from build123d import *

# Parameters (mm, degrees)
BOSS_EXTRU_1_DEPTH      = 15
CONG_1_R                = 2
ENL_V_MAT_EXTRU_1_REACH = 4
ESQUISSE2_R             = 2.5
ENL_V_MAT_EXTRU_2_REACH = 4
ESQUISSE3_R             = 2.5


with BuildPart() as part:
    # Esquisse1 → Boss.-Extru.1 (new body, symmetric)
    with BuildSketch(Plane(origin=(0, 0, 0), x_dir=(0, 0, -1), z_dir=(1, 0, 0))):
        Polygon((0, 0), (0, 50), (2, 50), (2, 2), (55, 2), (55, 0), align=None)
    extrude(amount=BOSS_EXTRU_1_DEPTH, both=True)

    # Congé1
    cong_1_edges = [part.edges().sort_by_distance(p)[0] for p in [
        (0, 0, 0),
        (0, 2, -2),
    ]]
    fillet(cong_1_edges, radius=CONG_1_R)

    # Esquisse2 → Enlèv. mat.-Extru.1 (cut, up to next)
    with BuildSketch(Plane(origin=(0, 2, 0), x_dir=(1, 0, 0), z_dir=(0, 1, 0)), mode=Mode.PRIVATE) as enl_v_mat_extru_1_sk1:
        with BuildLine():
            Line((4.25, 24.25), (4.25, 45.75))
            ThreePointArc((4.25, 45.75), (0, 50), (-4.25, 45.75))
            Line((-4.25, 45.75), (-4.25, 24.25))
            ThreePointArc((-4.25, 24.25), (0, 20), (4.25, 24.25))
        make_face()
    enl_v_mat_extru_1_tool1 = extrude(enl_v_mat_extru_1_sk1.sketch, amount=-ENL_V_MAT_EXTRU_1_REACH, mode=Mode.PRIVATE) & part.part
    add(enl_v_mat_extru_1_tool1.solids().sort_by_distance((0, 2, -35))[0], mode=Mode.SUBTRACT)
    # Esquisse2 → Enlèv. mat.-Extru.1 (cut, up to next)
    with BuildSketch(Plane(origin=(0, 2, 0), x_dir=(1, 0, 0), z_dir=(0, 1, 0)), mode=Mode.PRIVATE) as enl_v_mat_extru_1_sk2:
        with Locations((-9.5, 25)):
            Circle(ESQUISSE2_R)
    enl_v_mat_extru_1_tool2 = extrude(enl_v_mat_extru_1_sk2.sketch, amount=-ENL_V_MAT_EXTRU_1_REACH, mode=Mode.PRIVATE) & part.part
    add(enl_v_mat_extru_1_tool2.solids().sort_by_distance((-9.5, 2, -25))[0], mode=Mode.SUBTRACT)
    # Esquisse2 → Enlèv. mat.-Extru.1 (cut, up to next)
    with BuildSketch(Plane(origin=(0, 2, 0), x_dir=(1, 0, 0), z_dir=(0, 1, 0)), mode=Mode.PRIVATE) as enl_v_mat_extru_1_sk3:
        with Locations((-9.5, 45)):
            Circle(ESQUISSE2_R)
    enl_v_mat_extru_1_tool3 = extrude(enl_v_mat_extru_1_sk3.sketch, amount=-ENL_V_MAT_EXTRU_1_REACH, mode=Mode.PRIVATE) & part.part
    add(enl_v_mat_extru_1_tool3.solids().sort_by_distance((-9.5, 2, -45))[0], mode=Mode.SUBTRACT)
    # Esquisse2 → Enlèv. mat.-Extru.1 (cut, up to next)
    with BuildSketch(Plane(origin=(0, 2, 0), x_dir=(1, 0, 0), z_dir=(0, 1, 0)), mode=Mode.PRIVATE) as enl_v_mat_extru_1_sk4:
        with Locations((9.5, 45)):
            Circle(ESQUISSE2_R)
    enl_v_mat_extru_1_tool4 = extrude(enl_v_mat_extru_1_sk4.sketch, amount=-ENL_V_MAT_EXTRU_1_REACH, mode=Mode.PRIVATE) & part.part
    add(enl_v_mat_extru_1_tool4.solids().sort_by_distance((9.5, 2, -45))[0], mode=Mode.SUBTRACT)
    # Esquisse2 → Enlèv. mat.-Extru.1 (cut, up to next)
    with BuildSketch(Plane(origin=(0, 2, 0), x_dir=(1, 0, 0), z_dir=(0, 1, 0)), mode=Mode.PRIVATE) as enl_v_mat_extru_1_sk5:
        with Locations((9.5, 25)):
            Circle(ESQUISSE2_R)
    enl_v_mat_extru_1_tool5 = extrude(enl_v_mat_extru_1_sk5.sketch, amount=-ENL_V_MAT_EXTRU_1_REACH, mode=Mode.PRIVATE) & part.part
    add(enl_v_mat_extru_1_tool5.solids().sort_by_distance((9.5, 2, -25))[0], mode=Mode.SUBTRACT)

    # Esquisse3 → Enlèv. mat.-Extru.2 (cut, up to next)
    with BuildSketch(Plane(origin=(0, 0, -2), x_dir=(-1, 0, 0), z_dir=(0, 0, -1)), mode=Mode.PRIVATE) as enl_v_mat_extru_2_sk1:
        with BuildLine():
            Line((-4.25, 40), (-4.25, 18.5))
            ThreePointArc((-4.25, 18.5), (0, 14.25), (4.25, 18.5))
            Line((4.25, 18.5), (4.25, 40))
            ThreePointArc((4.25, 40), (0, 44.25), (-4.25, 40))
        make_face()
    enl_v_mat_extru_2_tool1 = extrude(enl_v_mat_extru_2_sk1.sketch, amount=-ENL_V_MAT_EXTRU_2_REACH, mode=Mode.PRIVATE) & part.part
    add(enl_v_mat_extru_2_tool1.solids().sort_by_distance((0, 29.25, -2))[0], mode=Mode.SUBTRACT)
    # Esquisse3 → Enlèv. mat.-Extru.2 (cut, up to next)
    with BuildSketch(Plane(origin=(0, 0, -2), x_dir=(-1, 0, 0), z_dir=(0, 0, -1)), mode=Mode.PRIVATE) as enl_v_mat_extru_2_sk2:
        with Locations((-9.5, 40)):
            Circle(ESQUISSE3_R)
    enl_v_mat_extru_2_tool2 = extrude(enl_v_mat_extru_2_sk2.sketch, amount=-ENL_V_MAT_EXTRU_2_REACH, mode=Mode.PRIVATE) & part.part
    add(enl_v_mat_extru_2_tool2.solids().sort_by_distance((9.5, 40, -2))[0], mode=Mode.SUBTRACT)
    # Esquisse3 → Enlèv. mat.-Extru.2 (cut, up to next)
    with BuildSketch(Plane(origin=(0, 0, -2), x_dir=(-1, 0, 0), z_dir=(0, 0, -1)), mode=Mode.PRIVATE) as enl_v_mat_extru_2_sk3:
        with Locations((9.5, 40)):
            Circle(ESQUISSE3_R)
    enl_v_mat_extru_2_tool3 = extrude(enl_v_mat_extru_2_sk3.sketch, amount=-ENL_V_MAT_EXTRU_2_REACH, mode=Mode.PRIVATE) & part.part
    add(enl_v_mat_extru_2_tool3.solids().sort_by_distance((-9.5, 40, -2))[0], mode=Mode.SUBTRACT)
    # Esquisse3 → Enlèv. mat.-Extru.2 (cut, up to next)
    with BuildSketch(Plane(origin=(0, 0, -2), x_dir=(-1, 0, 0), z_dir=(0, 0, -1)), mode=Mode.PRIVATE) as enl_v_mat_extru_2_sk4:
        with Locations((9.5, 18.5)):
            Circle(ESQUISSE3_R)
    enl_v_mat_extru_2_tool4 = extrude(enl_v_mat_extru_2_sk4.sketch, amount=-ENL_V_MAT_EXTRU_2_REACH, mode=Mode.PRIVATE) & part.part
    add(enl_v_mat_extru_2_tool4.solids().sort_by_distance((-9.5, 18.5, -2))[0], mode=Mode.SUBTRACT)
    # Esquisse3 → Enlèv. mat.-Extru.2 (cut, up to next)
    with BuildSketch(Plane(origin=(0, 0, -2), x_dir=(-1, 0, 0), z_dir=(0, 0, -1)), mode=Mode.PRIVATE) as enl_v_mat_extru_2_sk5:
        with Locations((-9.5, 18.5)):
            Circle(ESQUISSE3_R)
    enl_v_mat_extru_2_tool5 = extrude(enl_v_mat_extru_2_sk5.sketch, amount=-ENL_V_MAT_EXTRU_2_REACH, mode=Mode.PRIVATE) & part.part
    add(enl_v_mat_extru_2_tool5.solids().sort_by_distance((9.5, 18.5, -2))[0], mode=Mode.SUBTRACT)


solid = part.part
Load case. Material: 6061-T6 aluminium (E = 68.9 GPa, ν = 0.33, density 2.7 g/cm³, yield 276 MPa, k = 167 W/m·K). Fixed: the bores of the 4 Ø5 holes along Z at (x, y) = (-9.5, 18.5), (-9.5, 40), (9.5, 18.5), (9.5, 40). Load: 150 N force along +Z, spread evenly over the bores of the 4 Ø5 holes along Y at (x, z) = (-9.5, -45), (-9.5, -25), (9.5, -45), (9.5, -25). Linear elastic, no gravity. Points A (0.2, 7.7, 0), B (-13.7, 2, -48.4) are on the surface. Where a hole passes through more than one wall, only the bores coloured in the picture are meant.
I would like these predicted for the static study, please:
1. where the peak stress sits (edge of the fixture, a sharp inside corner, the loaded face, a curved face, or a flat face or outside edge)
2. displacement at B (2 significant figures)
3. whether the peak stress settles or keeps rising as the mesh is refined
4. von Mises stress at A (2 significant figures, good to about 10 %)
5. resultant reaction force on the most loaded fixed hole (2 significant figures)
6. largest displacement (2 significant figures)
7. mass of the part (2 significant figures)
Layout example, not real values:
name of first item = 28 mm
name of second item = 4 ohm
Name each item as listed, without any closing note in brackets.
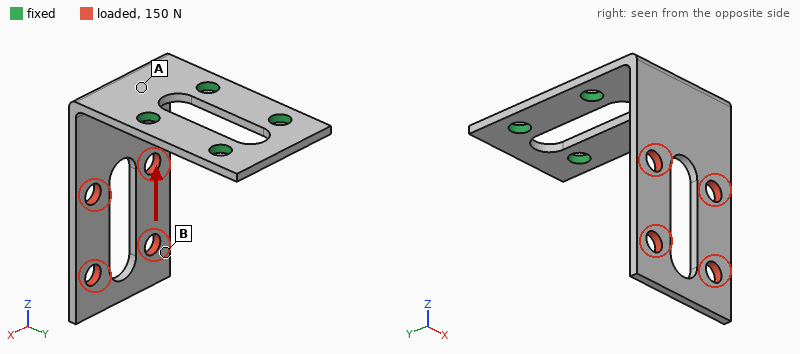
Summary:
where the peak stress sits = edge of the fixture
displacement at B = 0.69 mm
whether the peak stress settles or keeps rising as the mesh is refined = keeps rising
von Mises stress at A = 41 MPa
resultant reaction force on the most loaded fixed hole = 75 N
largest displacement = 0.79 mm
mass of the part = 13 g
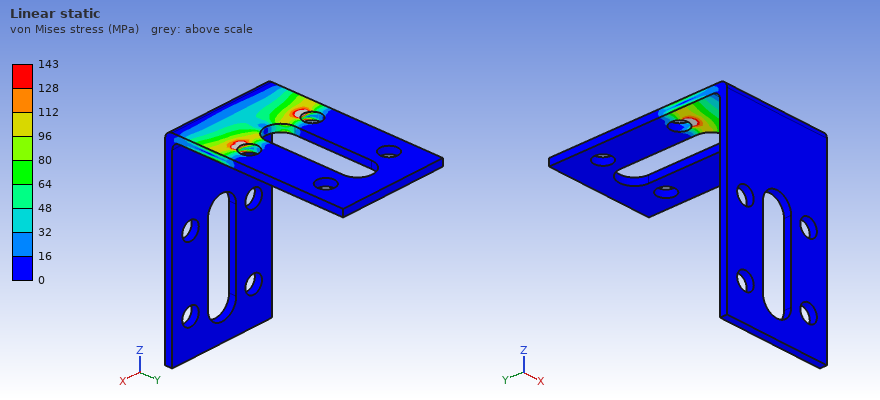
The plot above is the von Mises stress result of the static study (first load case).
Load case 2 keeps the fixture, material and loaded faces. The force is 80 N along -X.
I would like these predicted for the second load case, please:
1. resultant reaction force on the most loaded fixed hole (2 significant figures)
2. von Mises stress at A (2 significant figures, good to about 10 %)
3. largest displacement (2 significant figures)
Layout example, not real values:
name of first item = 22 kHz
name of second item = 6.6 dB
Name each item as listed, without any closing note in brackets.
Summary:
resultant reaction force on the most loaded fixed hole = 140 N
von Mises stress at A = 56 MPa
largest displacement = 0.48 mm
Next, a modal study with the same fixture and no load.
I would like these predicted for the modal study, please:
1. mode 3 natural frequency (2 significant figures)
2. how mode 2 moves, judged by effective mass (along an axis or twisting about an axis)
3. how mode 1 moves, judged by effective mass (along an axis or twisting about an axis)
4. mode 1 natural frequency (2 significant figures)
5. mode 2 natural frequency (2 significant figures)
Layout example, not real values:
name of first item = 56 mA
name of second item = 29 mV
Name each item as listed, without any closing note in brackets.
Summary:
mode 3 natural frequency = 1900 Hz
how mode 2 moves, judged by effective mass = along X
how mode 1 moves, judged by effective mass = along Y
mode 1 natural frequency = 440 Hz
mode 2 natural frequency = 1100 Hz
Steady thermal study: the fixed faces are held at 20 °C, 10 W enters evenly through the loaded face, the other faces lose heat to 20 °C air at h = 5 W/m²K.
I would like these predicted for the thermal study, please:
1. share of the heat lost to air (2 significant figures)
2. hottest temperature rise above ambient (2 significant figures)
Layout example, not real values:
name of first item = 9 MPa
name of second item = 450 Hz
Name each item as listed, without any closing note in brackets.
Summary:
share of the heat lost to air = 6.5 %
hottest temperature rise above ambient = 59 K
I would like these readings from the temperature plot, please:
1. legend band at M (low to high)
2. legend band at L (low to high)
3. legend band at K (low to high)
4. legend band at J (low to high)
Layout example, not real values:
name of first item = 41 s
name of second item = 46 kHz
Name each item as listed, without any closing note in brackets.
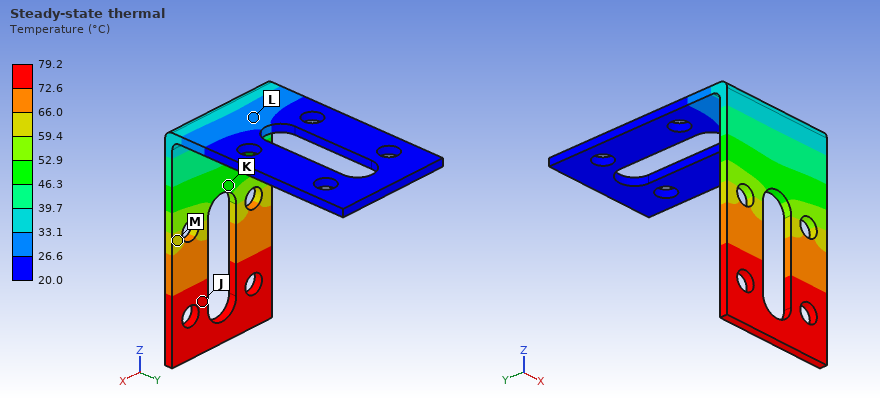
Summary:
legend band at M = 59.4 to 66.0 °C
legend band at L = 26.6 to 33.1 °C
legend band at K = 46.3 to 52.9 °C
legend band at J = 72.6 to 79.2 °C
